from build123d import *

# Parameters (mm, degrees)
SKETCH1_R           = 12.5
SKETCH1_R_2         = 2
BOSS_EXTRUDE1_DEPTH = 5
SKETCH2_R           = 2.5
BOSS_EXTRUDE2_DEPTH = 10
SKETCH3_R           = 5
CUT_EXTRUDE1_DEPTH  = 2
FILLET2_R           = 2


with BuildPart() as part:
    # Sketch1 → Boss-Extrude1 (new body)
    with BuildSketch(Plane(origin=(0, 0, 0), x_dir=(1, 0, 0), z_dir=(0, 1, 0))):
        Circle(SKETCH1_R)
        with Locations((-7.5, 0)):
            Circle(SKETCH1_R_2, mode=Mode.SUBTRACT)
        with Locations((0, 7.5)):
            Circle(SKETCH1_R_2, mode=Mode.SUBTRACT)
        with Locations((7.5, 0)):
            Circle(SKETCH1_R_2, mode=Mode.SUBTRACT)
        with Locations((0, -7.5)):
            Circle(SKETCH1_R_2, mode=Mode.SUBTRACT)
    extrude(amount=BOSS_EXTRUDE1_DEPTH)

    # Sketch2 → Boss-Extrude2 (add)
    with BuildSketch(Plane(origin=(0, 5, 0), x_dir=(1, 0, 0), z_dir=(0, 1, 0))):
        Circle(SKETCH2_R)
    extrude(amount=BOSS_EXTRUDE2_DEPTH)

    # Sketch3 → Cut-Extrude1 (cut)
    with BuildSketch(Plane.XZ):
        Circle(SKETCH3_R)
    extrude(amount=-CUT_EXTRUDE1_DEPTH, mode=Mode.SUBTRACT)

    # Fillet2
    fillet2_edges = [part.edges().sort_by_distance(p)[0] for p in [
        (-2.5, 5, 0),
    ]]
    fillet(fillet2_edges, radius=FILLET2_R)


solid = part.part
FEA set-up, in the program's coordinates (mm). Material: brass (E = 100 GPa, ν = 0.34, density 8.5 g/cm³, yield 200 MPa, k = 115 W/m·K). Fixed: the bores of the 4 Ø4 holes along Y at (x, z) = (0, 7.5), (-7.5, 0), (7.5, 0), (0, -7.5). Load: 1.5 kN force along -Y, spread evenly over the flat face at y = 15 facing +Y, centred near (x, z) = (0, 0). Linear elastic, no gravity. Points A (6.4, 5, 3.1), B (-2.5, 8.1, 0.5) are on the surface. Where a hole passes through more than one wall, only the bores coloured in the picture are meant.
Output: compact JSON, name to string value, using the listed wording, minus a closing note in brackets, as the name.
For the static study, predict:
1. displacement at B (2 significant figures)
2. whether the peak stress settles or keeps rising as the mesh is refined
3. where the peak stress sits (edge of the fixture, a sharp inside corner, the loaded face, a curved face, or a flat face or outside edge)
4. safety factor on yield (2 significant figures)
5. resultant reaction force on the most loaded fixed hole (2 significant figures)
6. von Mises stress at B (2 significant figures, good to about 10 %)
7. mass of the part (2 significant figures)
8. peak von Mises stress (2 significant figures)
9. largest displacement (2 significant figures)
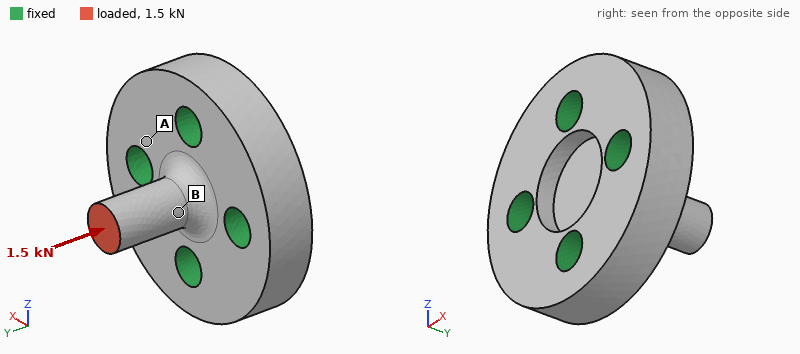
{"displacement at B": "4.9 µm", "whether the peak stress settles or keeps rising as the mesh is refined": "settles", "where the peak stress sits": "a curved face", "safety factor on yield": "1.9", "resultant reaction force on the most loaded fixed hole": "430 N", "von Mises stress at B": "75 MPa", "mass of the part": "19 g", "peak von Mises stress": "100 MPa", "largest displacement": "10 µm"}
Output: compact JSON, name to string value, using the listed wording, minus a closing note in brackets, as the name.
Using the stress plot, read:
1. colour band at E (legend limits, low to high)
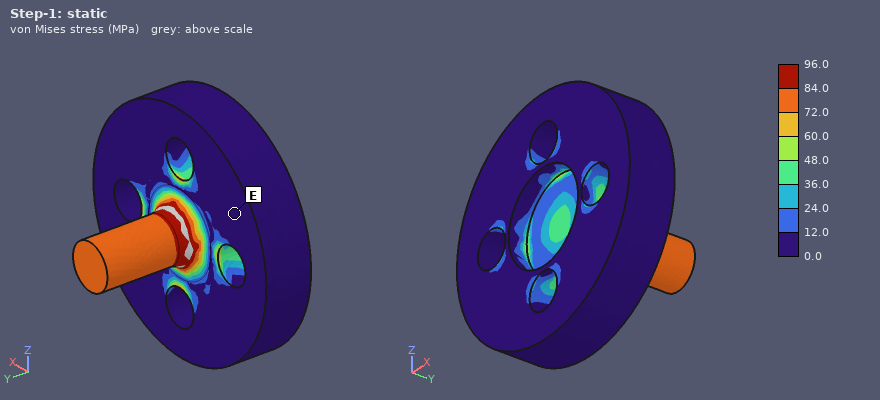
{"colour band at E": "0.0 to 12.0 MPa"}
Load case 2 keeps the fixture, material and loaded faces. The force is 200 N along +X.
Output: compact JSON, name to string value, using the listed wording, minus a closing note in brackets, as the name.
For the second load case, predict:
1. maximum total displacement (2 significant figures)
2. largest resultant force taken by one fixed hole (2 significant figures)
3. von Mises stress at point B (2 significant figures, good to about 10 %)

{"maximum total displacement": "27 µm", "largest resultant force taken by one fixed hole": "220 N", "von Mises stress at point B": "110 MPa"}
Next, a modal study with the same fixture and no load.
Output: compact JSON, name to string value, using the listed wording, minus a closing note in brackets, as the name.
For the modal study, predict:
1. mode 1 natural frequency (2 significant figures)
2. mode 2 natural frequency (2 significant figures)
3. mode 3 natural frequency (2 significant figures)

{"mode 1 natural frequency": "21 kHz", "mode 2 natural frequency": "21 kHz", "mode 3 natural frequency": "54 kHz"}
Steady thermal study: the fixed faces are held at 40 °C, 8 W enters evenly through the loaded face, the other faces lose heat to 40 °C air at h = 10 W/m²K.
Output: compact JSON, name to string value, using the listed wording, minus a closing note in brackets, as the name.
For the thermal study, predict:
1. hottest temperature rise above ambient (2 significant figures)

{"hottest temperature rise above ambient": "39 K"}
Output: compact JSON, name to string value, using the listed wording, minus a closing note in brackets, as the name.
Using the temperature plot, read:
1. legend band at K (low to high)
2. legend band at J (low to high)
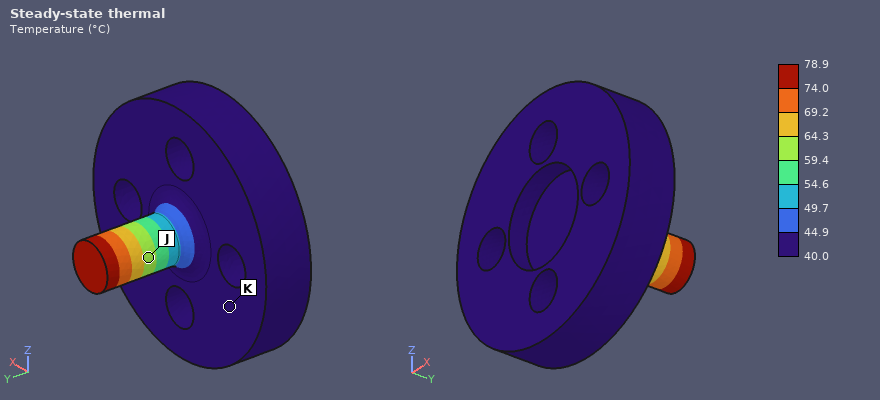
{"legend band at K": "40.0 to 44.9 °C", "legend band at J": "59.4 to 64.3 °C"}
